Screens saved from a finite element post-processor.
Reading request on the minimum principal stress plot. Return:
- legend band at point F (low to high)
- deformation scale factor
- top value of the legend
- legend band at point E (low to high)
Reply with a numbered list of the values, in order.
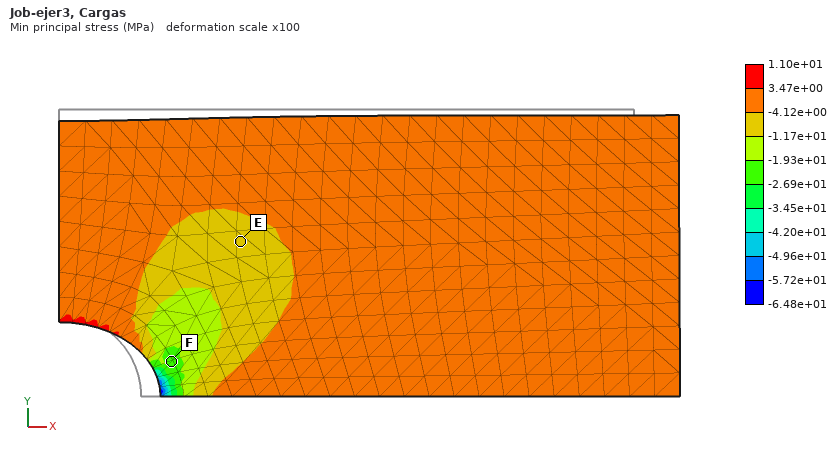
1. -2.69e+01 to -1.93e+01 MPa
2. 100
3. 1.10e+01 MPa
4. -1.17e+01 to -4.12e+00 MPa
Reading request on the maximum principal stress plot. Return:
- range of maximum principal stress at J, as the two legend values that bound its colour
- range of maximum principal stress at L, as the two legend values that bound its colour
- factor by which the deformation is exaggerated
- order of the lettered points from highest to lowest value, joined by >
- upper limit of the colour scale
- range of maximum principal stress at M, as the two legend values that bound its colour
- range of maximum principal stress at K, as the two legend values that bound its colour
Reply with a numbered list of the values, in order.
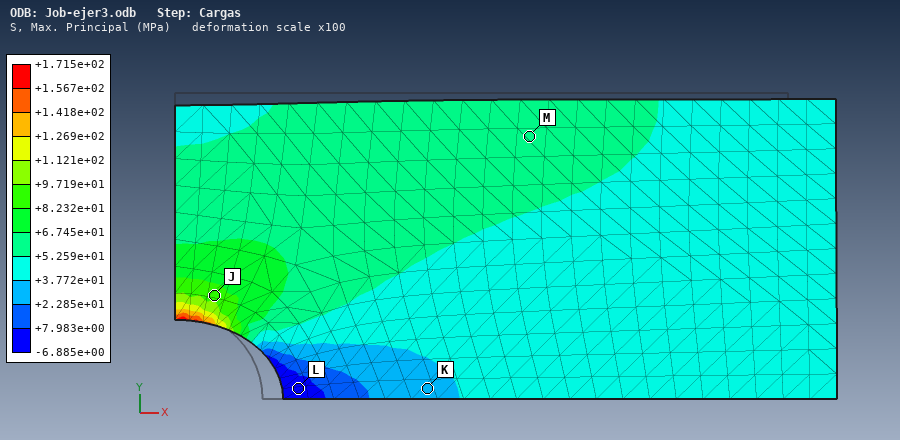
1. +8.232e+01 to +9.719e+01 MPa
2. -6.885e+00 to +7.983e+00 MPa
3. 100
4. J > M > K > L
5. +1.715e+02 MPa
6. +5.259e+01 to +6.745e+01 MPa
7. +2.285e+01 to +3.772e+01 MPa
